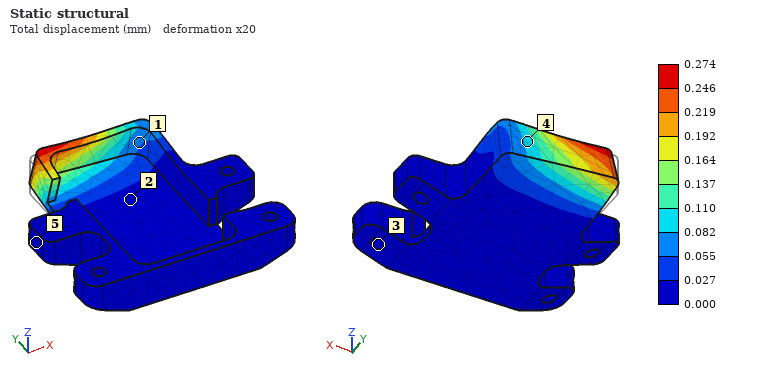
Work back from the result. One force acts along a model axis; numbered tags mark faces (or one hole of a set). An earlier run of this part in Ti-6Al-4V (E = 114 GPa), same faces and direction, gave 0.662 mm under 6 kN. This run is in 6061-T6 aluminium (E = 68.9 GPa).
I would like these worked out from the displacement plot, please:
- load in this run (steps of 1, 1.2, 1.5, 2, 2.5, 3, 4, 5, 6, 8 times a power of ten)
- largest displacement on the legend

1.5 kN
0.274 mm
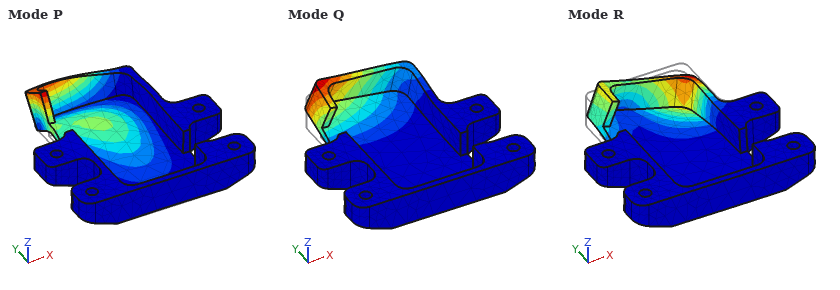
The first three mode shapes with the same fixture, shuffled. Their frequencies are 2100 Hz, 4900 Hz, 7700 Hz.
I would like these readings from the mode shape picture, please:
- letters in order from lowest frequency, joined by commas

Q, R, P
